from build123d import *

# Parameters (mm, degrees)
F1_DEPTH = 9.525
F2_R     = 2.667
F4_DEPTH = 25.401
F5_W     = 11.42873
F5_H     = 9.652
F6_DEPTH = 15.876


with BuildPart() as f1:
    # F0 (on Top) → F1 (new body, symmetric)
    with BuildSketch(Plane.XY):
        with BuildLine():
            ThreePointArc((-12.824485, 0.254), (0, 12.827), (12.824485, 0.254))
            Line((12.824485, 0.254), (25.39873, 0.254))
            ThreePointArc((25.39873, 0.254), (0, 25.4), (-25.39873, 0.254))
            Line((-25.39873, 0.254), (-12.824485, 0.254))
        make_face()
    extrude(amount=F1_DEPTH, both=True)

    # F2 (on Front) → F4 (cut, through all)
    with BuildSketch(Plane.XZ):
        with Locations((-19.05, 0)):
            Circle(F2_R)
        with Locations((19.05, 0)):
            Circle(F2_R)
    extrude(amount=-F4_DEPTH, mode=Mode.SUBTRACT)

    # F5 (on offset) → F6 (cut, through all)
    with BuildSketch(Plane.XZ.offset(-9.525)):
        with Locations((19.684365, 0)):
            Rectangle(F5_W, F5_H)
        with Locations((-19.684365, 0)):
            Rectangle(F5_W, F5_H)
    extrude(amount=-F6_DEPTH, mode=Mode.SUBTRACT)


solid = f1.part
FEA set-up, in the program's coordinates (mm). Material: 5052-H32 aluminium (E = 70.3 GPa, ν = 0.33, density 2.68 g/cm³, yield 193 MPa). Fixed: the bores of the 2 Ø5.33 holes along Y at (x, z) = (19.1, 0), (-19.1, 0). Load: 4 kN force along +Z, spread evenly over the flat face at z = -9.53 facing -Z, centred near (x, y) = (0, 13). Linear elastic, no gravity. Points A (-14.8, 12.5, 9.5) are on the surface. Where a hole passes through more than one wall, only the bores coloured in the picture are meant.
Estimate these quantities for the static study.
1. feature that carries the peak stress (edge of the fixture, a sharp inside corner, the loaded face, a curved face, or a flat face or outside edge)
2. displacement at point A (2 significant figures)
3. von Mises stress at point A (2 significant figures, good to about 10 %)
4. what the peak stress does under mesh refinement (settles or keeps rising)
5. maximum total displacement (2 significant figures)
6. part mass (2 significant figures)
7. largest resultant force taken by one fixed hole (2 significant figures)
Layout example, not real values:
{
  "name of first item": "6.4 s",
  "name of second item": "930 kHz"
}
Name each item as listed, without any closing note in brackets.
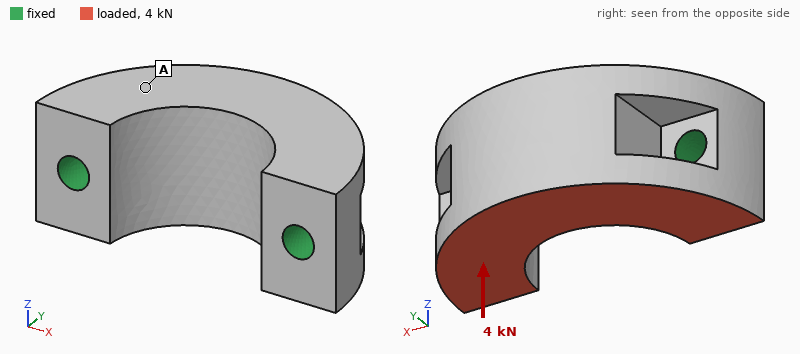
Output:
{
  "feature that carries the peak stress": "edge of the fixture",
  "displacement at point A": "13 µm",
  "von Mises stress at point A": "17 MPa",
  "what the peak stress does under mesh refinement": "keeps rising",
  "maximum total displacement": "30 µm",
  "part mass": "34 g",
  "largest resultant force taken by one fixed hole": "2.0 kN"
}
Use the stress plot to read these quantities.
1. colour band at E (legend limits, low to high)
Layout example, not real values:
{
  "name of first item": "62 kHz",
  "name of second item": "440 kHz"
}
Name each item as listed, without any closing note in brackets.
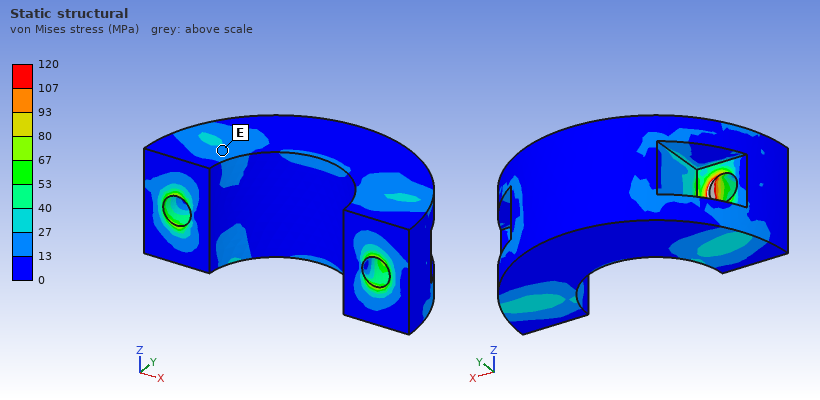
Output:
{
  "colour band at E": "13 to 27 MPa"
}
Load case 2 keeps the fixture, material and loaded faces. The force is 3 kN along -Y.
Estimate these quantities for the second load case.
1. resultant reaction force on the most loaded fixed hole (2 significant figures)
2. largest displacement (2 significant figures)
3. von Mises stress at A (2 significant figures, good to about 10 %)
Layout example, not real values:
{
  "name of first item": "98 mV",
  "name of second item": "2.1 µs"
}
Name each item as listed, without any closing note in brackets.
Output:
{
  "resultant reaction force on the most loaded fixed hole": "1.6 kN",
  "largest displacement": "22 µm",
  "von Mises stress at A": "13 MPa"
}
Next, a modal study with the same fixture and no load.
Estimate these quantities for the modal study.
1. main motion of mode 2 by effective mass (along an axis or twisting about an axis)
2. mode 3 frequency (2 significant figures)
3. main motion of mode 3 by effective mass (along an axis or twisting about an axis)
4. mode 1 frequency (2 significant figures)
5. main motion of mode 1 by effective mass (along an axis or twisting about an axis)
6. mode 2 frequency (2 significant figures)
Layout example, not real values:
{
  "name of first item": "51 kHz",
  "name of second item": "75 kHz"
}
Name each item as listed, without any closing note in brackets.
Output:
{
  "main motion of mode 2 by effective mass": "along X",
  "mode 3 frequency": "28 kHz",
  "main motion of mode 3 by effective mass": "along Y",
  "mode 1 frequency": "12 kHz",
  "main motion of mode 1 by effective mass": "along Z",
  "mode 2 frequency": "26 kHz"
}
